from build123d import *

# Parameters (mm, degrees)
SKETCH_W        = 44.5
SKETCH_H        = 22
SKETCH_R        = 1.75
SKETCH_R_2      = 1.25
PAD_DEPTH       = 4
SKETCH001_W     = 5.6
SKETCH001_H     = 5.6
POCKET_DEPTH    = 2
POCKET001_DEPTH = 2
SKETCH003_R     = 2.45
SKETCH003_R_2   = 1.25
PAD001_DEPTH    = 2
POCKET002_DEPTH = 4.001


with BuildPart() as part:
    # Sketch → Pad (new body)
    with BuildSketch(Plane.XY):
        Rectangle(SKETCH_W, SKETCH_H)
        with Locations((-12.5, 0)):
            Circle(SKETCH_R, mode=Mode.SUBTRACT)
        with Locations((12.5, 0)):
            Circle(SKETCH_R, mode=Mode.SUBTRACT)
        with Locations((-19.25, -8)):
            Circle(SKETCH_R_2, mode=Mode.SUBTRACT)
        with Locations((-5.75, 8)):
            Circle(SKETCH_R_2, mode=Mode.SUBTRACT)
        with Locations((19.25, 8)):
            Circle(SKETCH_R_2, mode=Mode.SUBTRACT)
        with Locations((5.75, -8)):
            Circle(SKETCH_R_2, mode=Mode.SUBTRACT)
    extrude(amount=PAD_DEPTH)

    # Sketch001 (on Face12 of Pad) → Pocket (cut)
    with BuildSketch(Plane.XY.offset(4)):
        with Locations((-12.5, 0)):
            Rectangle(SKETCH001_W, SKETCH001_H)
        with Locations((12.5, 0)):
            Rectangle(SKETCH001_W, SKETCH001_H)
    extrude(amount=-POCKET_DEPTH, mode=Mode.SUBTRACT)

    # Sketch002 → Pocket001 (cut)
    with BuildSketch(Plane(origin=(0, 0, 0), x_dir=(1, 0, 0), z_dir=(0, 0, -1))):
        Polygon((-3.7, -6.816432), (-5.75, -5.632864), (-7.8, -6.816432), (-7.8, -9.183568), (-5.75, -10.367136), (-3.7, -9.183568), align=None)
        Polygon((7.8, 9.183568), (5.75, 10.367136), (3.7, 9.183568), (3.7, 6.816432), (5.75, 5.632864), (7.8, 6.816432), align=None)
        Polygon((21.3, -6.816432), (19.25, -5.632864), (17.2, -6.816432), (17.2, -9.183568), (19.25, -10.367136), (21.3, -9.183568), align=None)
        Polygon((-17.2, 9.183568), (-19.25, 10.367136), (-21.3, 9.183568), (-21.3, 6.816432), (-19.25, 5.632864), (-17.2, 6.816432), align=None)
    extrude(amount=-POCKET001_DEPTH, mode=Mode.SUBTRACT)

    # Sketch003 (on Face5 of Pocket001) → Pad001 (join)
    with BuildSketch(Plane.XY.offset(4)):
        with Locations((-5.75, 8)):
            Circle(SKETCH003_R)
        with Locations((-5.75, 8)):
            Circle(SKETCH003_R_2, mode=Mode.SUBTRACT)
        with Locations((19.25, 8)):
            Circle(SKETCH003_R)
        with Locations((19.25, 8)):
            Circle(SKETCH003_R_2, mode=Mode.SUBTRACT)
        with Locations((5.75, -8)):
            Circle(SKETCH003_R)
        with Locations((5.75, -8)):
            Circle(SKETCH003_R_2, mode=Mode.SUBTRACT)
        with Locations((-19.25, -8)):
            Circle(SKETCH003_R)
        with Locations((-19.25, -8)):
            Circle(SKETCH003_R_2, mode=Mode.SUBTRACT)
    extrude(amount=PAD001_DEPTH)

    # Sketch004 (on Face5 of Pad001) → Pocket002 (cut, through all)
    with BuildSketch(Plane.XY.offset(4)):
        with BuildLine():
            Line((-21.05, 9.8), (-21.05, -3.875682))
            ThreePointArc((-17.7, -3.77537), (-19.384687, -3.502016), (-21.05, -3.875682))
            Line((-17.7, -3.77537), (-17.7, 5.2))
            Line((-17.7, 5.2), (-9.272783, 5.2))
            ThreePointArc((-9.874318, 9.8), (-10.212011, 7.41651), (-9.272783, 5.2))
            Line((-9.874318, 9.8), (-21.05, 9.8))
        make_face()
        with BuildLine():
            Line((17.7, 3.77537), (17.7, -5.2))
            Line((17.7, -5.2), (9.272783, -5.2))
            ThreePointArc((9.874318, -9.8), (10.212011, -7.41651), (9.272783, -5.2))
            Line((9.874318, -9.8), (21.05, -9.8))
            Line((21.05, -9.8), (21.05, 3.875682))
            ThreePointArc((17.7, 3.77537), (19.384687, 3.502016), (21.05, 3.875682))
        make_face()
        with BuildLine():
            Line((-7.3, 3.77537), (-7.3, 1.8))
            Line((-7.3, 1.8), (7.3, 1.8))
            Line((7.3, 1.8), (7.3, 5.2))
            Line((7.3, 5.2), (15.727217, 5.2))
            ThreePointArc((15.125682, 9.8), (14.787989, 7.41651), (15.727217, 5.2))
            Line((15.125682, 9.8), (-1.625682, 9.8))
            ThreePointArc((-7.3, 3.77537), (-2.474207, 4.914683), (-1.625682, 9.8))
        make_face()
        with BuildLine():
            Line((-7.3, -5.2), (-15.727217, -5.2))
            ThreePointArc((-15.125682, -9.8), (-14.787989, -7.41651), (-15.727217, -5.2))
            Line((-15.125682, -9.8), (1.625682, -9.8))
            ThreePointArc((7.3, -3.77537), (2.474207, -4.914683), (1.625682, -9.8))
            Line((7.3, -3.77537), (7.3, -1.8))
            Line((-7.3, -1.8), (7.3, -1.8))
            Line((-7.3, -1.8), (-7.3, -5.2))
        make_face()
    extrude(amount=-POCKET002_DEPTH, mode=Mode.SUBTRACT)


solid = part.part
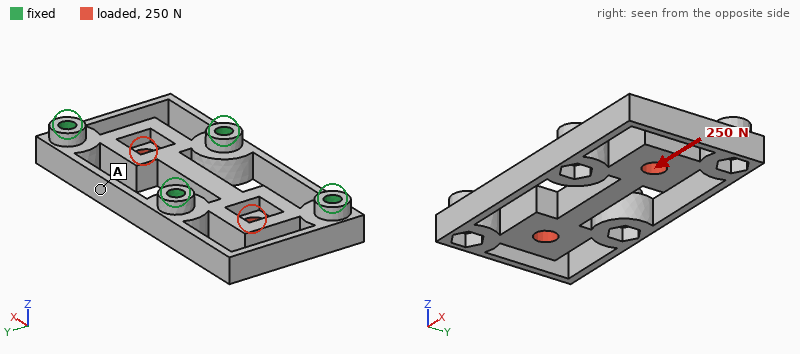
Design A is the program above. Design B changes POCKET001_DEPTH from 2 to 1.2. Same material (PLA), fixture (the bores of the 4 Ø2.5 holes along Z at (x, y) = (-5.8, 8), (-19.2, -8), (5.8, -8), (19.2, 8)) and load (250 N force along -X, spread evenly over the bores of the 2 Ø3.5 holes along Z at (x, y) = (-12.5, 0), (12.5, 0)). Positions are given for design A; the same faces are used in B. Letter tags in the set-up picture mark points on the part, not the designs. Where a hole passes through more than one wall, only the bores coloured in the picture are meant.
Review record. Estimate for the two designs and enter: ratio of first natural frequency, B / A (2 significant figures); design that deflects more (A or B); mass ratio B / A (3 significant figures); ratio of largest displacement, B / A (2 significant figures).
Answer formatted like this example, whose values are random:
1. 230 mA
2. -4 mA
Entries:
1. 1.1
2. A
3. 1.01
4. 0.87
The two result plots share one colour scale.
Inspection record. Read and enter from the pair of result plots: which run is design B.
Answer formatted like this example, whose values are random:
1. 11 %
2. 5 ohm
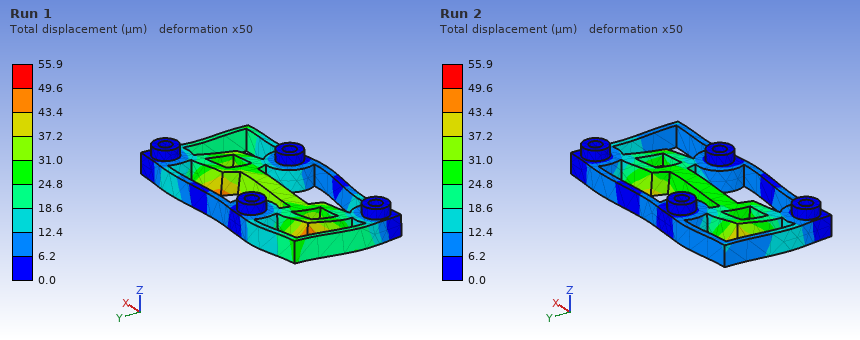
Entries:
1. Run 2
